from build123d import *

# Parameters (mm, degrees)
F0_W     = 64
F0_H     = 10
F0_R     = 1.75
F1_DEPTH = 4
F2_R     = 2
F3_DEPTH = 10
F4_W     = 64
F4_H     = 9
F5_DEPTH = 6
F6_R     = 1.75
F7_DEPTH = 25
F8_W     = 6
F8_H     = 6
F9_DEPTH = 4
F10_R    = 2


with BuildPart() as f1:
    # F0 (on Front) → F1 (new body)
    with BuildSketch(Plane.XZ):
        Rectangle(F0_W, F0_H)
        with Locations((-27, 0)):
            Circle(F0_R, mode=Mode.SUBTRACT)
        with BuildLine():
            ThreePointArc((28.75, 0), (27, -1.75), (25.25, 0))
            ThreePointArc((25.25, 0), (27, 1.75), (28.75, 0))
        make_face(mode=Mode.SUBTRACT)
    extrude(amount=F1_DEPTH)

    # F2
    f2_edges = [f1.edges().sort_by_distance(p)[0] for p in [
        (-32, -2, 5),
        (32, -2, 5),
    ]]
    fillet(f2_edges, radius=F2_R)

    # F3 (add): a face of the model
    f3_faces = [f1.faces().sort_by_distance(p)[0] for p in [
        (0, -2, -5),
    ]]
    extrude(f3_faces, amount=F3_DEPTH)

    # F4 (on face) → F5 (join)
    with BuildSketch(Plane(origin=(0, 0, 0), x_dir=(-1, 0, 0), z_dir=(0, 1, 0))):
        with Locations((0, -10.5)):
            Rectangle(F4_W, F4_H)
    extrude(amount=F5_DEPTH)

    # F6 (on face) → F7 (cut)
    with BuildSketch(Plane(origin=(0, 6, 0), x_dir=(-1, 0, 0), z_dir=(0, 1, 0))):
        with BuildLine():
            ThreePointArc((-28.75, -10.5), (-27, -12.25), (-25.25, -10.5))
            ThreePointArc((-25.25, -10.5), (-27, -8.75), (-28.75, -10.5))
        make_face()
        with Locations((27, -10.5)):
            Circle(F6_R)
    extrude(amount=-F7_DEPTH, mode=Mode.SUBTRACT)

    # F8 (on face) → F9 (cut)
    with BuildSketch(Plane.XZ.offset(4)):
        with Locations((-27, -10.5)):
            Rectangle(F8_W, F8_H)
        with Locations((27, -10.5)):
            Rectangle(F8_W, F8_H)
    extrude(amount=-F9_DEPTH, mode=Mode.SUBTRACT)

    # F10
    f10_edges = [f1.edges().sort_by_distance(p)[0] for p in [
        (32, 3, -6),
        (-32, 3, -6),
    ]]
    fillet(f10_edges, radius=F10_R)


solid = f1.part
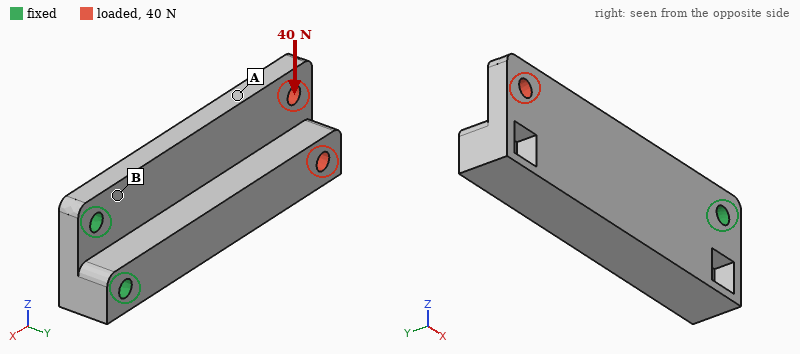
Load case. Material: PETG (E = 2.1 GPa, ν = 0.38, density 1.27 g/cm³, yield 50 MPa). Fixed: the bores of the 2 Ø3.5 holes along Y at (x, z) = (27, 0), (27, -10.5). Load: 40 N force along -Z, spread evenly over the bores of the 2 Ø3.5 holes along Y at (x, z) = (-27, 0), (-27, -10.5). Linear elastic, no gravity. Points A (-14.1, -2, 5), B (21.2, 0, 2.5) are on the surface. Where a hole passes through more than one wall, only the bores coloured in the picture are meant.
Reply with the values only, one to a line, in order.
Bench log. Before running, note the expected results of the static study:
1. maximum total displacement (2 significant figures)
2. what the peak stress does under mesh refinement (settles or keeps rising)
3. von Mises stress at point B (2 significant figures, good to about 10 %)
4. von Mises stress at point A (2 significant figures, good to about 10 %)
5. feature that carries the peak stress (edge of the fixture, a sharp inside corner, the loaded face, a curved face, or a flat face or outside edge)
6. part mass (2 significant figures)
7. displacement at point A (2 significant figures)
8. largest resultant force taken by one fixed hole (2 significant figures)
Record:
0.72 mm
keeps rising
6.8 MPa
1.7 MPa
edge of the fixture
10 g
0.39 mm
140 N
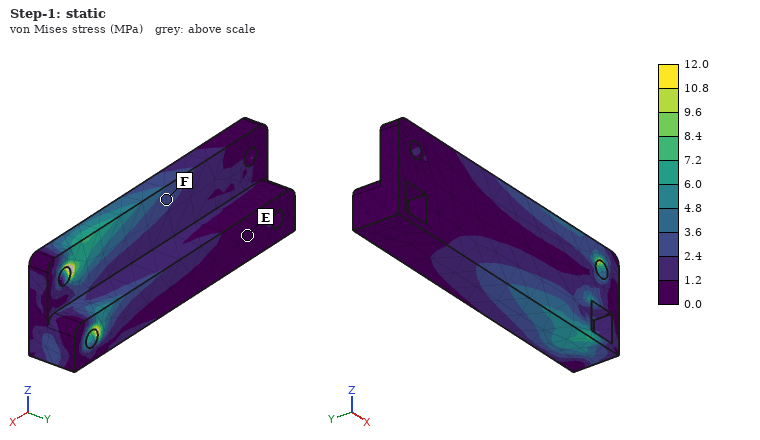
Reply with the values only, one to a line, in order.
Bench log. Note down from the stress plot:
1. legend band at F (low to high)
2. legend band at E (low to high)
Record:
2.4 to 3.6 MPa
0.0 to 1.2 MPa
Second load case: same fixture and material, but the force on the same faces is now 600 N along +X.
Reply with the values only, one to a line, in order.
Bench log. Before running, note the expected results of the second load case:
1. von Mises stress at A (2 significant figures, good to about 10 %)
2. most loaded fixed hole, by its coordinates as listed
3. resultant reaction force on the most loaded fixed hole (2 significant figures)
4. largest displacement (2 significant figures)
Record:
6.8 MPa
(27, -10.5)
370 N
0.67 mm
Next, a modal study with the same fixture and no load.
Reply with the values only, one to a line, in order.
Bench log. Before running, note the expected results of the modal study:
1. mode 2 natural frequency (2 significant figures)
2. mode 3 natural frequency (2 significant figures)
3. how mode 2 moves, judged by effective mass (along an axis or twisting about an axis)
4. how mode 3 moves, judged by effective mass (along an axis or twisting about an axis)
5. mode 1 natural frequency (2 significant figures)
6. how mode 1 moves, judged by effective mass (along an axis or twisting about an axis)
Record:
1000 Hz
1900 Hz
along Z
twisting about X
450 Hz
along Y
